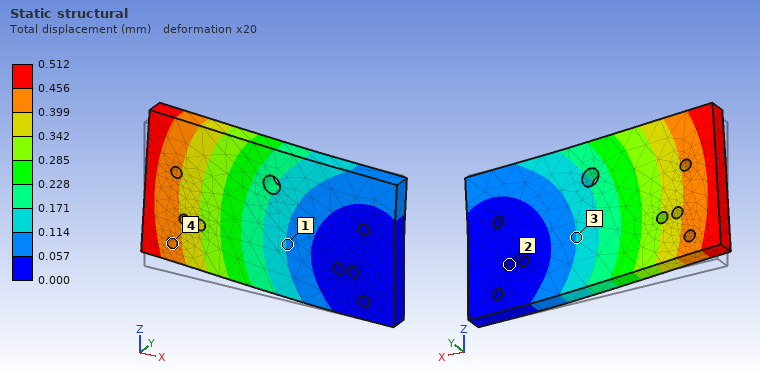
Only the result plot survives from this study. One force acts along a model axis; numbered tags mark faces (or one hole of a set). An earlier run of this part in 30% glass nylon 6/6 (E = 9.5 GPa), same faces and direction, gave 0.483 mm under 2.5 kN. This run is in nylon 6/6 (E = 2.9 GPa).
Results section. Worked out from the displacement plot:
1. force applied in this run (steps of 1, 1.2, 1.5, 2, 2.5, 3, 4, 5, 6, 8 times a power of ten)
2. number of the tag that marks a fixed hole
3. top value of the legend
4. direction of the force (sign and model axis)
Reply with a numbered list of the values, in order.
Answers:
1. 800 N
2. 2
3. 0.512 mm
4. +Z
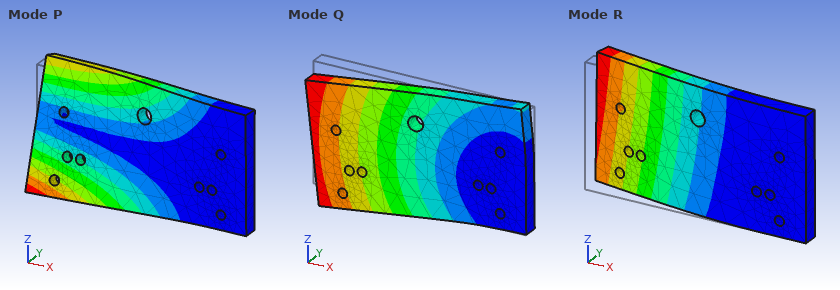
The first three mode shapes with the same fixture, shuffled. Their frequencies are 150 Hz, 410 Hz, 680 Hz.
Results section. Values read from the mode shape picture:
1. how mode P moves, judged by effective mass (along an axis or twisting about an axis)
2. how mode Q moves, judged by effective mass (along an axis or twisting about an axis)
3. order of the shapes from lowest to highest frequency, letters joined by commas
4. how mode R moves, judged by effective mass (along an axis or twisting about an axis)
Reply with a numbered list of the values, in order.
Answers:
1. twisting about X
2. along Z
3. R, P, Q
4. along Y
